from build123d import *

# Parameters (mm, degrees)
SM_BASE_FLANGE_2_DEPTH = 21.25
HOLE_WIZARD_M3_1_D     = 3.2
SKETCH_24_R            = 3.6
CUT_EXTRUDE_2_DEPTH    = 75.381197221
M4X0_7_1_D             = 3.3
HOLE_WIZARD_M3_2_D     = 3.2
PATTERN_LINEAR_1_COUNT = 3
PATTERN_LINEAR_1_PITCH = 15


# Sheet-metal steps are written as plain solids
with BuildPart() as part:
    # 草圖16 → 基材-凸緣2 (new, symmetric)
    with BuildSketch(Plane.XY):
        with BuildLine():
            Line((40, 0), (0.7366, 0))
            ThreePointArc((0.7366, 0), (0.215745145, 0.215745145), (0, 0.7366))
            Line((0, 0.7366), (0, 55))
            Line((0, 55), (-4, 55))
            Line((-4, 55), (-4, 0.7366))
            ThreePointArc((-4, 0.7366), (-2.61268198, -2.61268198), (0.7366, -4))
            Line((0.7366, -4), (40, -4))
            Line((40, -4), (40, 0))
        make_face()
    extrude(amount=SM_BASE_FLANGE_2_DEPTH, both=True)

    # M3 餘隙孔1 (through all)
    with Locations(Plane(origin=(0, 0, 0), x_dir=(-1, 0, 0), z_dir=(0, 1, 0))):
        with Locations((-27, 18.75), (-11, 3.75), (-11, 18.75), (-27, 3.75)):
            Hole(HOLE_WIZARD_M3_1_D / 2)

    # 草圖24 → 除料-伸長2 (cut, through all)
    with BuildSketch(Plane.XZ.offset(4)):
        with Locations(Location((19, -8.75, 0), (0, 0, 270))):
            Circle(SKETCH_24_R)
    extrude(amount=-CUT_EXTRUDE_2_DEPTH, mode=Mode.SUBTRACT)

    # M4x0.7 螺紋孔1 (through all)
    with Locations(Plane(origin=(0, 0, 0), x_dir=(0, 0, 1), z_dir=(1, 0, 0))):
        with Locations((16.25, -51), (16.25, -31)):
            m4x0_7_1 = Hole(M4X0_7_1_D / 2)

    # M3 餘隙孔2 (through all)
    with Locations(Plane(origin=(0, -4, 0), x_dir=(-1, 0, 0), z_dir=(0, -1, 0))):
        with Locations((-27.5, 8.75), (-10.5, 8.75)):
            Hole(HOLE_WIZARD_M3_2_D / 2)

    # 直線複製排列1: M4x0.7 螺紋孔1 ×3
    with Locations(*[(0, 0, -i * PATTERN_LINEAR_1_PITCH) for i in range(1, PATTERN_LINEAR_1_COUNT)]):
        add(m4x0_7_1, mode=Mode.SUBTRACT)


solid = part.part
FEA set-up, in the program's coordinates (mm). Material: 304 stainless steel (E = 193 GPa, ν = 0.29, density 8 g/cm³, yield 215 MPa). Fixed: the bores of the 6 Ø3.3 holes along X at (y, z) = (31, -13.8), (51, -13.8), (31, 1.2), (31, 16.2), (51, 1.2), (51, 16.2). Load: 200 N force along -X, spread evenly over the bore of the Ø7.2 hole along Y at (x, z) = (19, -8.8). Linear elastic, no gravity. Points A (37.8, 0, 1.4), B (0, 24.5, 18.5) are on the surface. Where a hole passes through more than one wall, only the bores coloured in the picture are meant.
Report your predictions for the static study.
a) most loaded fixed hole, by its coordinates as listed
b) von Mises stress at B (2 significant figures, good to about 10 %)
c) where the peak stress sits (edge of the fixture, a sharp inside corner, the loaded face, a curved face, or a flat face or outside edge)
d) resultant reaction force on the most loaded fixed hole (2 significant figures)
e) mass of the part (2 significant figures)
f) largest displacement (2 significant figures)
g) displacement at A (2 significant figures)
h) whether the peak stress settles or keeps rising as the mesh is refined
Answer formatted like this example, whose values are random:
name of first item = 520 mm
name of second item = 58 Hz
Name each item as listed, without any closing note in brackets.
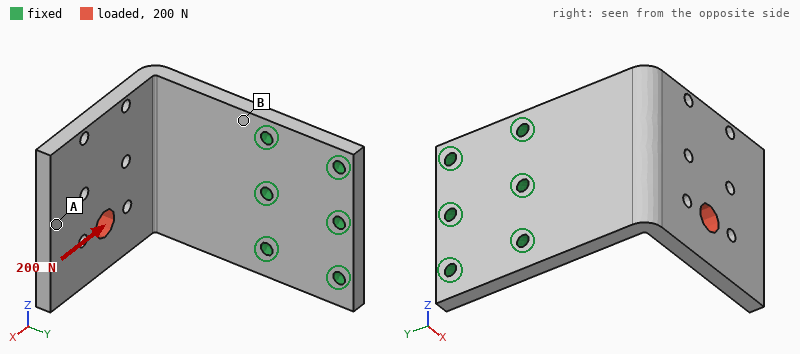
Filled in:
most loaded fixed hole, by its coordinates as listed = (31, -13.8)
von Mises stress at B = 37 MPa
where the peak stress sits = edge of the fixture
resultant reaction force on the most loaded fixed hole = 140 N
mass of the part = 130 g
largest displacement = 0.13 mm
displacement at A = 0.11 mm
whether the peak stress settles or keeps rising as the mesh is refined = keeps rising
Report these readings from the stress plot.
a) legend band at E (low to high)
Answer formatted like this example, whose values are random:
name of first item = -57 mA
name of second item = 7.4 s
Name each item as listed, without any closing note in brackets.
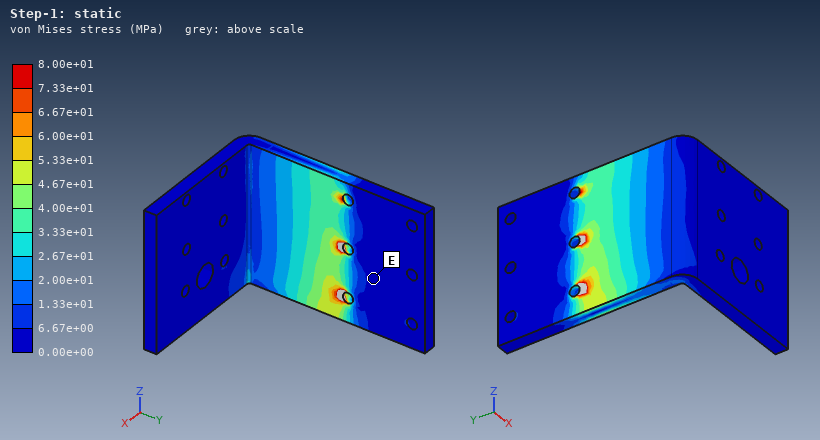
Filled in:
legend band at E = 0.00e+00 to 6.67e+00 MPa
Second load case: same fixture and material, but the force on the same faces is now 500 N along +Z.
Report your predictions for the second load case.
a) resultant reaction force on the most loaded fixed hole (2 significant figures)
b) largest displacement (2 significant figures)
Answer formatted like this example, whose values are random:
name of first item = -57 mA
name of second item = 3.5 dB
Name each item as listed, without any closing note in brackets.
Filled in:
resultant reaction force on the most loaded fixed hole = 600 N
largest displacement = 0.15 mm
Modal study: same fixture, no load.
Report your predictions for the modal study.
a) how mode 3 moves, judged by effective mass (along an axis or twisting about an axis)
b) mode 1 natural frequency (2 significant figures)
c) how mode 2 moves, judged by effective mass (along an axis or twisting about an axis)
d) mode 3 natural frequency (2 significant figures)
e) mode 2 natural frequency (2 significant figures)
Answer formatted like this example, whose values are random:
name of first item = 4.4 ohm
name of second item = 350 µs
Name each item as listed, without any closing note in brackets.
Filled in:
how mode 3 moves, judged by effective mass = along X
mode 1 natural frequency = 780 Hz
how mode 2 moves, judged by effective mass = along Z
mode 3 natural frequency = 2200 Hz
mode 2 natural frequency = 1400 Hz
